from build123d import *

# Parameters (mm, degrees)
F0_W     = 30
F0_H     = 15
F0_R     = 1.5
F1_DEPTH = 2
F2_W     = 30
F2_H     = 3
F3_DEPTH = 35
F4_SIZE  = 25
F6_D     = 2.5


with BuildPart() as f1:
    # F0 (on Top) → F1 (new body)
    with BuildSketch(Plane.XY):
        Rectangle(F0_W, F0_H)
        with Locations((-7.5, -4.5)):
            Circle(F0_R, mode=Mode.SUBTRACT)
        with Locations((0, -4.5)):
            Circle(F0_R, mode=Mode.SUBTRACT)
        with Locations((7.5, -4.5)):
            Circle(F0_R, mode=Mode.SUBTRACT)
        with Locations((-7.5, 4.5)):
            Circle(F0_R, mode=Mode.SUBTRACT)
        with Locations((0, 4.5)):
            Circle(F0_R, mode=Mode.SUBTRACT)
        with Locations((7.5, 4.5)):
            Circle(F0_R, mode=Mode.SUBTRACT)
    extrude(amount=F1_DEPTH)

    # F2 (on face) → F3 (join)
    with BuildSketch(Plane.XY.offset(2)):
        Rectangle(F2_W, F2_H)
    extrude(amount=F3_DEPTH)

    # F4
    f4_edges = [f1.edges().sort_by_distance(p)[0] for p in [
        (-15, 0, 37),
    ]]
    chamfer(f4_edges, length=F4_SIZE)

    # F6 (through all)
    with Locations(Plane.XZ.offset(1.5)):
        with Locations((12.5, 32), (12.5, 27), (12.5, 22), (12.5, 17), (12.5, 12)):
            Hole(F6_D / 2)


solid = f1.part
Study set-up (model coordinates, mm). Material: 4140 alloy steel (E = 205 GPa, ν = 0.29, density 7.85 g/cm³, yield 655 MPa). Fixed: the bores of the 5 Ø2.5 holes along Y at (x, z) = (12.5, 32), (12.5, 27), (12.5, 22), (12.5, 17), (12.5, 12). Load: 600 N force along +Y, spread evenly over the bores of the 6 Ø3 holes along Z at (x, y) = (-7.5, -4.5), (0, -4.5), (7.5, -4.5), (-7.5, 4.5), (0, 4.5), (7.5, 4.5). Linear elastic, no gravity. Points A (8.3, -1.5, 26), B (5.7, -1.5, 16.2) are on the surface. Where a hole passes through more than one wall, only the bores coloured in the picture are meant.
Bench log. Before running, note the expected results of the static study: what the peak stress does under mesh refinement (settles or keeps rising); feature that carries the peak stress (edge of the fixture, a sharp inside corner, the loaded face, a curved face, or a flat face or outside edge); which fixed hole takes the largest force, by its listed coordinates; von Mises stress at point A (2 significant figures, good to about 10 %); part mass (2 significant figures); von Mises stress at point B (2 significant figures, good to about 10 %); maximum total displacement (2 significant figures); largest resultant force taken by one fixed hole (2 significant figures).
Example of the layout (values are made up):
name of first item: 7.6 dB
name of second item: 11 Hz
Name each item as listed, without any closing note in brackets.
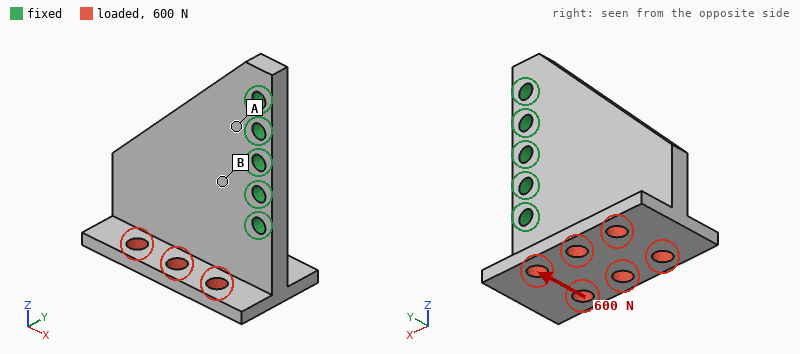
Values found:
what the peak stress does under mesh refinement: keeps rising
feature that carries the peak stress: edge of the fixture
which fixed hole takes the largest force, by its listed coordinates: (12.5, 12)
von Mises stress at point A: 52 MPa
part mass: 23 g
von Mises stress at point B: 160 MPa
maximum total displacement: 0.21 mm
largest resultant force taken by one fixed hole: 840 N
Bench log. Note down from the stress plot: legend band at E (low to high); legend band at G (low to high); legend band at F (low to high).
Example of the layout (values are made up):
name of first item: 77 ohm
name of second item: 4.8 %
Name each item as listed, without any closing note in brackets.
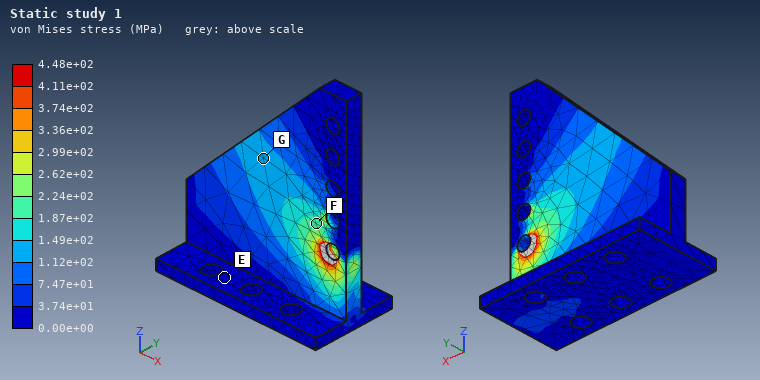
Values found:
legend band at E: 0.00e+00 to 3.74e+01 MPa
legend band at G: 1.12e+02 to 1.49e+02 MPa
legend band at F: 1.87e+02 to 2.24e+02 MPa
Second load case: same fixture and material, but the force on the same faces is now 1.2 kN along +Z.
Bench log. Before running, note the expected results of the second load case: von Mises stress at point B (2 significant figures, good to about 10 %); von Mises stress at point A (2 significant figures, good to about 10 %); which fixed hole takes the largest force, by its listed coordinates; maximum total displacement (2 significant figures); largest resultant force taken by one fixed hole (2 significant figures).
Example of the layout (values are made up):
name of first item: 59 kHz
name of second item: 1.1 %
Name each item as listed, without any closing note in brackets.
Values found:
von Mises stress at point B: 33 MPa
von Mises stress at point A: 30 MPa
which fixed hole takes the largest force, by its listed coordinates: (12.5, 12)
maximum total displacement: 15 µm
largest resultant force taken by one fixed hole: 790 N
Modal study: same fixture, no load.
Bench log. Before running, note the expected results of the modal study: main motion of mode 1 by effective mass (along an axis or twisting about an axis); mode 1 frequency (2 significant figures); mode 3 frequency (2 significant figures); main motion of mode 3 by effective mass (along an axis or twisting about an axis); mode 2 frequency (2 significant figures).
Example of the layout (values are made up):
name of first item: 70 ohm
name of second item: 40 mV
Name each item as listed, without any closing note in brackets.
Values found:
main motion of mode 1 by effective mass: along Y
mode 1 frequency: 3000 Hz
mode 3 frequency: 13 kHz
main motion of mode 3 by effective mass: along Y
mode 2 frequency: 7800 Hz
